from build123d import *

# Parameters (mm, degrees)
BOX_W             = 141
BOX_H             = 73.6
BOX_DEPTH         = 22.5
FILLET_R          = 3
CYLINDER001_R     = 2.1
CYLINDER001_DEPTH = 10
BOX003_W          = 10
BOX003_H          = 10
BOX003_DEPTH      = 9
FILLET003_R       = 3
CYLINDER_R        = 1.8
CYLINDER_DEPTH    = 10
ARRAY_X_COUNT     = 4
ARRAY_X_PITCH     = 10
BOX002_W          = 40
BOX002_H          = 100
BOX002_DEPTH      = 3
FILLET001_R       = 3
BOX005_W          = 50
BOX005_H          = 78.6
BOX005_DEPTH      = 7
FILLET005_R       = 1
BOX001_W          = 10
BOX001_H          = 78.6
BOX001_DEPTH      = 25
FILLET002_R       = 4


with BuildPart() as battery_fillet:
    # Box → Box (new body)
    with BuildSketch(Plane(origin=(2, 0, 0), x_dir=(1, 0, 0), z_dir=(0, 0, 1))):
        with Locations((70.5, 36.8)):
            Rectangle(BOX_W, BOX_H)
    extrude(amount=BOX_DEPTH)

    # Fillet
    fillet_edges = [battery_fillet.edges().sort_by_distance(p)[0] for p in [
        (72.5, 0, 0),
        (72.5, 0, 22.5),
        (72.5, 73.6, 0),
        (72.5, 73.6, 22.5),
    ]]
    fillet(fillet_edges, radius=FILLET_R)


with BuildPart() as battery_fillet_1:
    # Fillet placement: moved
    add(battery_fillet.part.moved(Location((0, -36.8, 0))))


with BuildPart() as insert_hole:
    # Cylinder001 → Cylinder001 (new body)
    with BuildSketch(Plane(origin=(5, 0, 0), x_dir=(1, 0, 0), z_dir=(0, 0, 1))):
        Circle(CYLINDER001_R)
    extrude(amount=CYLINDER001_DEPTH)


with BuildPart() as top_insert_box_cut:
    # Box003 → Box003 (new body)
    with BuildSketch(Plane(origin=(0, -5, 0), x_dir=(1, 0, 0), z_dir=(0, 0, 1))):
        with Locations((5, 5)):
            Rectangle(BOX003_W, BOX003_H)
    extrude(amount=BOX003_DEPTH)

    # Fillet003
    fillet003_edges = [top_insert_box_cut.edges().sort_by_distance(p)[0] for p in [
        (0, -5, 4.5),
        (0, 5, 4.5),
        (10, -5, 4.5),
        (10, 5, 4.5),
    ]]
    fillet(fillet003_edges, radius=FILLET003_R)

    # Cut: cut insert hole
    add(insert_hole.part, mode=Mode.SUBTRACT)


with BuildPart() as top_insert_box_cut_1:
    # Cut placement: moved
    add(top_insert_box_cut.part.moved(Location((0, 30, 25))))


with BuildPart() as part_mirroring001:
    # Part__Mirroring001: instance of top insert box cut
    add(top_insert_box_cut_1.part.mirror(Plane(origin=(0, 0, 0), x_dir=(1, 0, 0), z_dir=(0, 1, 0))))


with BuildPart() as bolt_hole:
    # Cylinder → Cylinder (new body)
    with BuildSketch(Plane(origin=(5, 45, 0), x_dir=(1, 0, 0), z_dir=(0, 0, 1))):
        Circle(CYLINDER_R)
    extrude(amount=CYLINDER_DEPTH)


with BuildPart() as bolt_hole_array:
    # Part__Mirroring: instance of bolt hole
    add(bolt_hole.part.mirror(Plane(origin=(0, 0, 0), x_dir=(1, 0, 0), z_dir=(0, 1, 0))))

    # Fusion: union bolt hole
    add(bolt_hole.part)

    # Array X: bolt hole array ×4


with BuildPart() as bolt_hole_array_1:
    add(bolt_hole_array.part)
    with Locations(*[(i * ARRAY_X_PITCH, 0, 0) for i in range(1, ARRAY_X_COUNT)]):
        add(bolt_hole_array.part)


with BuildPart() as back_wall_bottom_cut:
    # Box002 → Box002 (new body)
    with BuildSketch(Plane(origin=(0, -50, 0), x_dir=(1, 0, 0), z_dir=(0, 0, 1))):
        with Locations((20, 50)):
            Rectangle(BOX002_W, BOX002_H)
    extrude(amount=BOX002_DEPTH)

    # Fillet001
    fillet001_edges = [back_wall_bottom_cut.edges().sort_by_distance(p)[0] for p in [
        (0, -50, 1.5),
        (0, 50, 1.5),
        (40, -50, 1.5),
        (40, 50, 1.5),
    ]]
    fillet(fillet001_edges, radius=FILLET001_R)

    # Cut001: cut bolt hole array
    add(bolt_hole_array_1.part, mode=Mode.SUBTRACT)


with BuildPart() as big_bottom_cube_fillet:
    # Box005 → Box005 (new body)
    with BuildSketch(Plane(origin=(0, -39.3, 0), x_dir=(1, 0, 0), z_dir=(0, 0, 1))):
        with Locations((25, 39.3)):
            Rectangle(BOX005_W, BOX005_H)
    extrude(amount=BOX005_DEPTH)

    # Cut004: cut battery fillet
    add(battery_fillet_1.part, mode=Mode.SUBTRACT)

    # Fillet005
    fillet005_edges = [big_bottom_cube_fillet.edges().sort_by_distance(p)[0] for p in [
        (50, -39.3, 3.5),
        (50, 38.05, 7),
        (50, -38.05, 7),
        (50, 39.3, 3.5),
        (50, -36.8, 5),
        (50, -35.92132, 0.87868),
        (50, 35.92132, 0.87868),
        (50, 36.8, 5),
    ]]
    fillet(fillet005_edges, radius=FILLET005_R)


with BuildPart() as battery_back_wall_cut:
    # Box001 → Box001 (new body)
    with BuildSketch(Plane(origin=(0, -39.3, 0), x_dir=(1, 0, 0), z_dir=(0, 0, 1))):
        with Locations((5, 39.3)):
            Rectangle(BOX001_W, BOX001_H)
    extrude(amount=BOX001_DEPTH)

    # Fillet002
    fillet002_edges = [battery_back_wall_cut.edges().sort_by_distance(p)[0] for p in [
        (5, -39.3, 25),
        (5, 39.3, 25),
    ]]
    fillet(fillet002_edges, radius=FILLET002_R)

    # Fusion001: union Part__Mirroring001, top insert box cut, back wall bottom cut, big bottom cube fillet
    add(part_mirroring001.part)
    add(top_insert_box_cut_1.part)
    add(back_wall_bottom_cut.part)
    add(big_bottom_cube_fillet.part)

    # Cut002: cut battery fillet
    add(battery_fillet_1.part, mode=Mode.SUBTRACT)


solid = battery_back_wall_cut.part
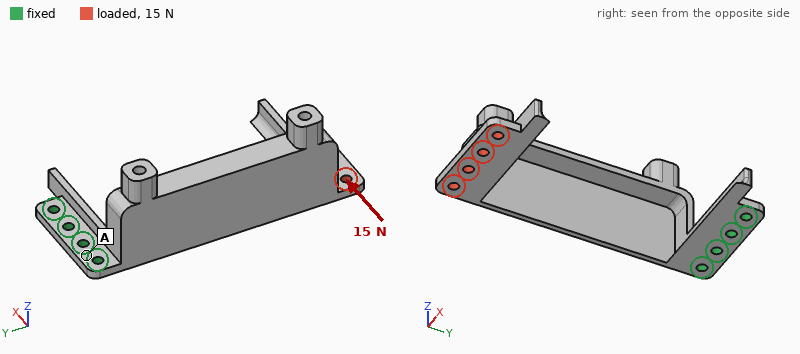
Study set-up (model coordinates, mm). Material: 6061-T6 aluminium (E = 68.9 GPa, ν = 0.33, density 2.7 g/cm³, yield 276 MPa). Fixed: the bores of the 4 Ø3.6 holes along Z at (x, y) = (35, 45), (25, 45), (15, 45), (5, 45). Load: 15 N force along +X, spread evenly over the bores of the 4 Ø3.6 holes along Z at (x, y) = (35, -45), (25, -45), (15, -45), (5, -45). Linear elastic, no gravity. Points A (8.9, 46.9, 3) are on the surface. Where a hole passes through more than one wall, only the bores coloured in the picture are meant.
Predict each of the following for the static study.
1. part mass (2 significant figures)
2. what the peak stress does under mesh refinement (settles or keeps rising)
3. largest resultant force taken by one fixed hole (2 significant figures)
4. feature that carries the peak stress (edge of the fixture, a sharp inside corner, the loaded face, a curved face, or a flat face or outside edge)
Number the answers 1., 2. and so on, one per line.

1. 31 g
2. keeps rising
3. 110 N
4. a sharp inside corner
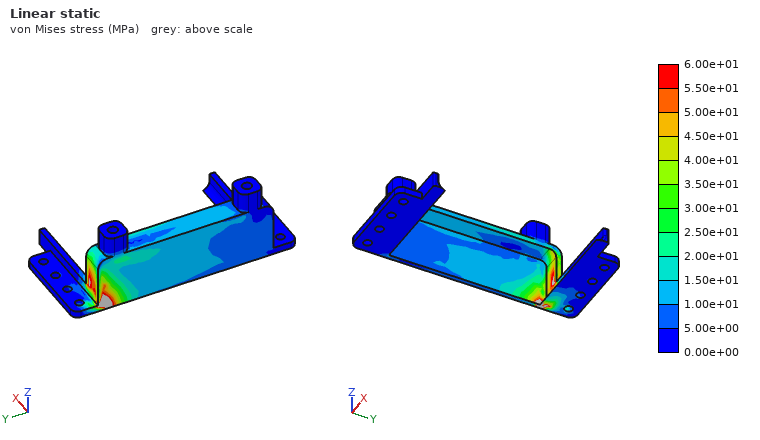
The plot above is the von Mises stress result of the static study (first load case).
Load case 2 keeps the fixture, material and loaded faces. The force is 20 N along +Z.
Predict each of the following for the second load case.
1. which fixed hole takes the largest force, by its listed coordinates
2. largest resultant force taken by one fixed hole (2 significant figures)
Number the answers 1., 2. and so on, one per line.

1. (15, 45)
2. 47 N
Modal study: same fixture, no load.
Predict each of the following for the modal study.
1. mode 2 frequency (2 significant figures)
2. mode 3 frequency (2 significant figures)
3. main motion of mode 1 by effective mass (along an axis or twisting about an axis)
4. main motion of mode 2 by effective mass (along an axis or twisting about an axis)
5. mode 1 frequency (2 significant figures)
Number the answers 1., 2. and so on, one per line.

1. 250 Hz
2. 600 Hz
3. along X
4. along Z
5. 190 Hz
